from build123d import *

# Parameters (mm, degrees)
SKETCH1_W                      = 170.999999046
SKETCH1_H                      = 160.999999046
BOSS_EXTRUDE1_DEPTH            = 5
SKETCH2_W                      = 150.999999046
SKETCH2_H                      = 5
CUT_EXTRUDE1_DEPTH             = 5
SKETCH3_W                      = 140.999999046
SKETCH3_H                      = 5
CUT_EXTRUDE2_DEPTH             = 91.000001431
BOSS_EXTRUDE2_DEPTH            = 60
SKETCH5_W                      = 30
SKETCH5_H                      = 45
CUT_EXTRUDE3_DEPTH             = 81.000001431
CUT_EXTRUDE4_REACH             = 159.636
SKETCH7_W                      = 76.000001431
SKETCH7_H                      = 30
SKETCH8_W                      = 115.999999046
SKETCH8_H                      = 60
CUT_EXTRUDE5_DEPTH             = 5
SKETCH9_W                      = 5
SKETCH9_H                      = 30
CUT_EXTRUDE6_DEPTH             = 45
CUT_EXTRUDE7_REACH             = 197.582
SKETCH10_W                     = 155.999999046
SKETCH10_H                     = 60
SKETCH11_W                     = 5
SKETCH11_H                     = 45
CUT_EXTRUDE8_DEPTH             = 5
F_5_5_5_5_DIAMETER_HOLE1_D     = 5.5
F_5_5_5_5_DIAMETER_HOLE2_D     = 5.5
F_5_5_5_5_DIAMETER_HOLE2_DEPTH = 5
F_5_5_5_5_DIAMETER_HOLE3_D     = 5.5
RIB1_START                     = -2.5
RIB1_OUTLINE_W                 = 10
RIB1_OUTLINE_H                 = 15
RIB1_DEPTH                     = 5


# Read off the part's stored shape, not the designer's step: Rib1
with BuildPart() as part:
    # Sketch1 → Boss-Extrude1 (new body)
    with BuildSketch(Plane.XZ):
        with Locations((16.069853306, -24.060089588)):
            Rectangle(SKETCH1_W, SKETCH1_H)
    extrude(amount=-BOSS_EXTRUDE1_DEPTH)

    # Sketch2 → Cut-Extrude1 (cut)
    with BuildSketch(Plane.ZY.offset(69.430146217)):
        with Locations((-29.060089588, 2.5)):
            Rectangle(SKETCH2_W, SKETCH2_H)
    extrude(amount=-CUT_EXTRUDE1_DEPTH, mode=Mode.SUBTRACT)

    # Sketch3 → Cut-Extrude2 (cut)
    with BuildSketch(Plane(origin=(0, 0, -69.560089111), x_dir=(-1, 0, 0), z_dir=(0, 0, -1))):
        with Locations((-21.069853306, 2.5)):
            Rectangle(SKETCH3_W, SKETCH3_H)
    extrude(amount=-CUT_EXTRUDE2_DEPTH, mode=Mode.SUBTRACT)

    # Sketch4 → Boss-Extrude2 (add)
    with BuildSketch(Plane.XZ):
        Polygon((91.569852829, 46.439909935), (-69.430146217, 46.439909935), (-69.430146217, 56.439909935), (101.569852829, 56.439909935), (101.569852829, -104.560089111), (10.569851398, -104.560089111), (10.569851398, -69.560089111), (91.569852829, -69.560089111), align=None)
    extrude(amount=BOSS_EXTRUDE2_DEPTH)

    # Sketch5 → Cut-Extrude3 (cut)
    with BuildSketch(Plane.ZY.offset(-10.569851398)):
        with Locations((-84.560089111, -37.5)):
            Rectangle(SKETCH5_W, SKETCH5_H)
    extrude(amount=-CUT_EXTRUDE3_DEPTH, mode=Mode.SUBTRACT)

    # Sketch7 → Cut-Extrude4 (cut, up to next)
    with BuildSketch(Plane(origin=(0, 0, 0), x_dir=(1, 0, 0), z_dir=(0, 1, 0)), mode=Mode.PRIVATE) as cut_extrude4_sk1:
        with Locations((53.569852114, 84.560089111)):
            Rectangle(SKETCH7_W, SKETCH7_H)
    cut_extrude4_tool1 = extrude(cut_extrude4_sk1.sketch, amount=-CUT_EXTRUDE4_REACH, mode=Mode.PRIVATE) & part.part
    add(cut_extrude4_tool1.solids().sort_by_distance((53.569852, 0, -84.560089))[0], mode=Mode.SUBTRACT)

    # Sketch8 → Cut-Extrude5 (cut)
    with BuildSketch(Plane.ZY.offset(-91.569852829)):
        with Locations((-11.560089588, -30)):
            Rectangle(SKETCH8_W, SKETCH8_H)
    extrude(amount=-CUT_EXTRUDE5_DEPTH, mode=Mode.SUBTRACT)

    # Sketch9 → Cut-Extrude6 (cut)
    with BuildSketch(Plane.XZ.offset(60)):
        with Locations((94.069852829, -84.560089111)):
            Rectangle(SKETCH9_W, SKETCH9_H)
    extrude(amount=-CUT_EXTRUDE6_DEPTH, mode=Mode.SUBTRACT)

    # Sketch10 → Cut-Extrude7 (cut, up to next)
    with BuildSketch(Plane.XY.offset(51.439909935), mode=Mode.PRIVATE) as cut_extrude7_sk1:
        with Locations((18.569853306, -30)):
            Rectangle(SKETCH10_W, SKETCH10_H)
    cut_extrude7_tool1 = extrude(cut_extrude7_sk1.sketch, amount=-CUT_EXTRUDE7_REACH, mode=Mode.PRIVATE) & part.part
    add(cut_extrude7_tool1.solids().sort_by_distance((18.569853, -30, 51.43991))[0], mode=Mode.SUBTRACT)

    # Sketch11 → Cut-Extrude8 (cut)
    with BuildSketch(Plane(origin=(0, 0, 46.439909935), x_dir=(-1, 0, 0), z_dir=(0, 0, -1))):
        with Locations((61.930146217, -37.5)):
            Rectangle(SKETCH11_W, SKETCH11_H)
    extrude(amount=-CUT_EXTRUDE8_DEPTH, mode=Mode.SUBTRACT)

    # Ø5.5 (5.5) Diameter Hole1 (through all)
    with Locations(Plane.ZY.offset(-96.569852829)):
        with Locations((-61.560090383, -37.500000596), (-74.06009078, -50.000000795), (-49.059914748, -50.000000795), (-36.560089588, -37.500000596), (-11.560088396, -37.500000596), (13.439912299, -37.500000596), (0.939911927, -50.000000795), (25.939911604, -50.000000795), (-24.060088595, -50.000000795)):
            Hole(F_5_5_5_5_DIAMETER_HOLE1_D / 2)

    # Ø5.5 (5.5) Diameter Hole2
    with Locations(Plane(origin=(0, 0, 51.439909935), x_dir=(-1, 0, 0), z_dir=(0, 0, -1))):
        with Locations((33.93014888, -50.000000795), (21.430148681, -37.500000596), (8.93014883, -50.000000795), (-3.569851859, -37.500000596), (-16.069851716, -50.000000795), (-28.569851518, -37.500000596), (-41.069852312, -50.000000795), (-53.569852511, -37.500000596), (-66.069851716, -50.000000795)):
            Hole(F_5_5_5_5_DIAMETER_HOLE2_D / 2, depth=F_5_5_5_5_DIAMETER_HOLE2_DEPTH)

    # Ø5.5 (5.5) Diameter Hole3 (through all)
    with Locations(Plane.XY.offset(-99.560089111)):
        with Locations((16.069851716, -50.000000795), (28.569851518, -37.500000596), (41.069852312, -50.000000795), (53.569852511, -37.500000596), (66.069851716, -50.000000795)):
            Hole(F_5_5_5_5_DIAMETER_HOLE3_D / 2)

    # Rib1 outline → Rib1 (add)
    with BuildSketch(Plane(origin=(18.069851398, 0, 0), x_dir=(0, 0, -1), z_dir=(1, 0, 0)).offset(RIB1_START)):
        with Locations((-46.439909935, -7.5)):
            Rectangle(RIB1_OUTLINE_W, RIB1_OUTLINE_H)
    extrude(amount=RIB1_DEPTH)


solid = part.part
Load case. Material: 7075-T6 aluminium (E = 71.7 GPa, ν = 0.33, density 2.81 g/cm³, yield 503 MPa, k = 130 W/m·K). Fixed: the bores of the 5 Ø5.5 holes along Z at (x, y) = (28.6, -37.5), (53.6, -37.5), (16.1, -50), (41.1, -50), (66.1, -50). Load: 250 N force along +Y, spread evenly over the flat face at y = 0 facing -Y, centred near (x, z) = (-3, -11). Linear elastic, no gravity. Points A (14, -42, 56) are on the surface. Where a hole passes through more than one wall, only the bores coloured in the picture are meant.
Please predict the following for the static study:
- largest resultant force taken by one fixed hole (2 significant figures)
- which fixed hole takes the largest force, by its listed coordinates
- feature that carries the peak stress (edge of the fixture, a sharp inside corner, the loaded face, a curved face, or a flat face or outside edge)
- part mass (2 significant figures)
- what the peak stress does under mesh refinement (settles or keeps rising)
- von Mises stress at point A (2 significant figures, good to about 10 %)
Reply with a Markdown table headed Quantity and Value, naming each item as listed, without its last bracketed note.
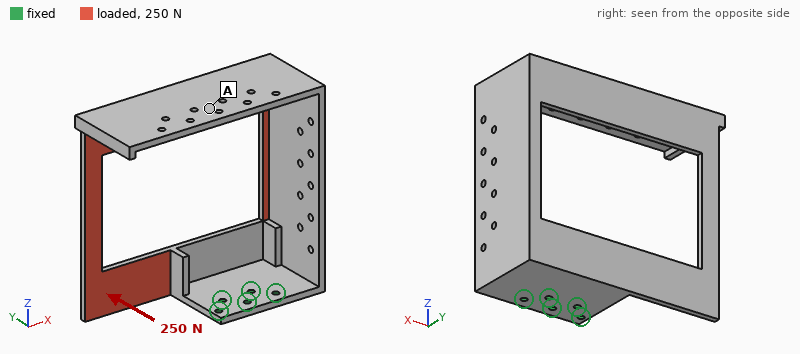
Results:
| Quantity | Value |
|---|---|
| largest resultant force taken by one fixed hole | 790 N |
| which fixed hole takes the largest force, by its listed coordinates | (53.6, -37.5) |
| feature that carries the peak stress | edge of the fixture |
| part mass | 560 g |
| what the peak stress does under mesh refinement | keeps rising |
| von Mises stress at point A | 4.3 MPa |
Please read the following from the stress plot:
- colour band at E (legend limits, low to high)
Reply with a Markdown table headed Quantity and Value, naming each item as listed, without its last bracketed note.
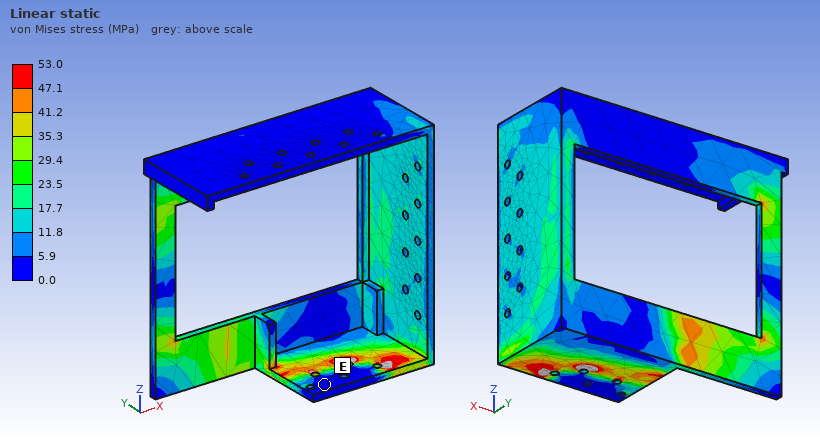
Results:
| Quantity | Value |
|---|---|
| colour band at E | 0.0 to 5.9 MPa |
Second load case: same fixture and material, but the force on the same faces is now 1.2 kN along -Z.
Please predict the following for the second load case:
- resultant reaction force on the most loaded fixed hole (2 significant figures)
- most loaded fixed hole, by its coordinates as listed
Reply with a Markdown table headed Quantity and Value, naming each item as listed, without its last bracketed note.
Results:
| Quantity | Value |
|---|---|
| resultant reaction force on the most loaded fixed hole | 2.2 kN |
| most loaded fixed hole, by its coordinates as listed | (28.6, -37.5) |
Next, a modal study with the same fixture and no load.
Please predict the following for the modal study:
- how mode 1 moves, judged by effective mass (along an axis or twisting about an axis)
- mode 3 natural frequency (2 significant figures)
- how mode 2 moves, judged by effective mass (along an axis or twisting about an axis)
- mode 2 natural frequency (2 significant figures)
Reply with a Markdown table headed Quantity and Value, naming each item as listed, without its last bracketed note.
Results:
| Quantity | Value |
|---|---|
| how mode 1 moves, judged by effective mass | along Y |
| mode 3 natural frequency | 280 Hz |
| how mode 2 moves, judged by effective mass | along X |
| mode 2 natural frequency | 110 Hz |
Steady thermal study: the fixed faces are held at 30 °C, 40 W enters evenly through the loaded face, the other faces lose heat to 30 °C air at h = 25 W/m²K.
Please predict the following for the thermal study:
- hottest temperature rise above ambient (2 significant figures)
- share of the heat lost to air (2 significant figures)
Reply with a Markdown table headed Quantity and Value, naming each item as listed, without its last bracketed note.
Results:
| Quantity | Value |
|---|---|
| hottest temperature rise above ambient | 38 K |
| share of the heat lost to air | 73 % |
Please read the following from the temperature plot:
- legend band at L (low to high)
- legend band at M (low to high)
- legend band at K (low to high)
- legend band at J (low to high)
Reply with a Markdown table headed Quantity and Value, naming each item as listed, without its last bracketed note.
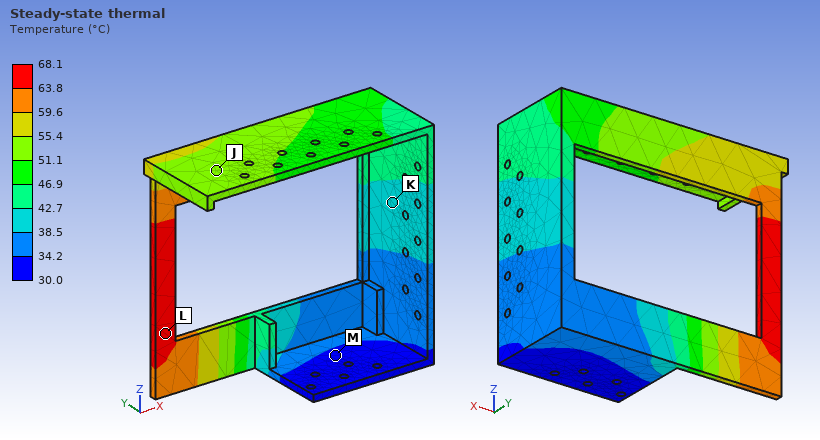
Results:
| Quantity | Value |
|---|---|
| legend band at L | 63.8 to 68.1 °C |
| legend band at M | 30.0 to 34.2 °C |
| legend band at K | 38.5 to 42.7 °C |
| legend band at J | 51.1 to 55.4 °C |
